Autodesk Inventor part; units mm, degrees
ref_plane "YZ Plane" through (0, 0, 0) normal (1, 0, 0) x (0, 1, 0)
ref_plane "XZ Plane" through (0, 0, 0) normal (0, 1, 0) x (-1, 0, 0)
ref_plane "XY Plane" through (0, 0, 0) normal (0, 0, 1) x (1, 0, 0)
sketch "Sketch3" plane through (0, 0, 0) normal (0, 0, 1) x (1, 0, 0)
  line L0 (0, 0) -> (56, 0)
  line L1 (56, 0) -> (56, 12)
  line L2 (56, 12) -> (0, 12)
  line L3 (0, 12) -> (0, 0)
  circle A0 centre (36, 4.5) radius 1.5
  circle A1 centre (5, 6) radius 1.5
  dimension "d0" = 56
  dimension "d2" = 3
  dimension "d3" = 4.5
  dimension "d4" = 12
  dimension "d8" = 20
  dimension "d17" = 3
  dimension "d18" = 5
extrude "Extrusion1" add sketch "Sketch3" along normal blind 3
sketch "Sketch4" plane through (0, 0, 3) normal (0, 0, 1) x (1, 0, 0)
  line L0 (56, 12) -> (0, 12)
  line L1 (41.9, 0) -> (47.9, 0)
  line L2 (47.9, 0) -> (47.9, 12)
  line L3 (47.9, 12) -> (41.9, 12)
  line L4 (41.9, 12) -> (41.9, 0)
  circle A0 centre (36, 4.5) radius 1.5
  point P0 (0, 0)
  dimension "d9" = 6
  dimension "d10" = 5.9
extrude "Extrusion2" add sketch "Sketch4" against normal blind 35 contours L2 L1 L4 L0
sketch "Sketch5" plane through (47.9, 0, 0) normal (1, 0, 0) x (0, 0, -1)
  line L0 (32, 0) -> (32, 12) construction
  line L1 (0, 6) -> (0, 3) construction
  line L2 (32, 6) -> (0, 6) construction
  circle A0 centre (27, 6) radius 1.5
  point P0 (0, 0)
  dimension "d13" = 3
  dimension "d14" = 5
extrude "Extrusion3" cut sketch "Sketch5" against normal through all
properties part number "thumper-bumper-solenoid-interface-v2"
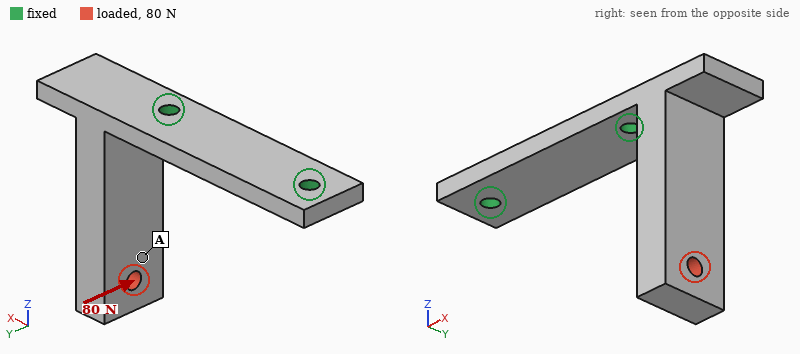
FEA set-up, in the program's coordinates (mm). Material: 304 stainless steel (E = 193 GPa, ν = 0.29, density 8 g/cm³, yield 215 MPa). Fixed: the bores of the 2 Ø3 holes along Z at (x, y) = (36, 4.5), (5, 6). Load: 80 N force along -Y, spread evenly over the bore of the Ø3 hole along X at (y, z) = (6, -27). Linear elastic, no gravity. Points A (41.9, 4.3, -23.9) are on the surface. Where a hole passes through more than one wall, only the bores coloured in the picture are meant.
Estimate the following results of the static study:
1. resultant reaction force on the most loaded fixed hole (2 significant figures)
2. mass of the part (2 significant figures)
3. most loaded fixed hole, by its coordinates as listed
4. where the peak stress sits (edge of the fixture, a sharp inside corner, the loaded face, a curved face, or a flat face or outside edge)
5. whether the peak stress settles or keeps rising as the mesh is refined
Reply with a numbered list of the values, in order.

1. 94 N
2. 34 g
3. (36, 4.5)
4. edge of the fixture
5. keeps rising
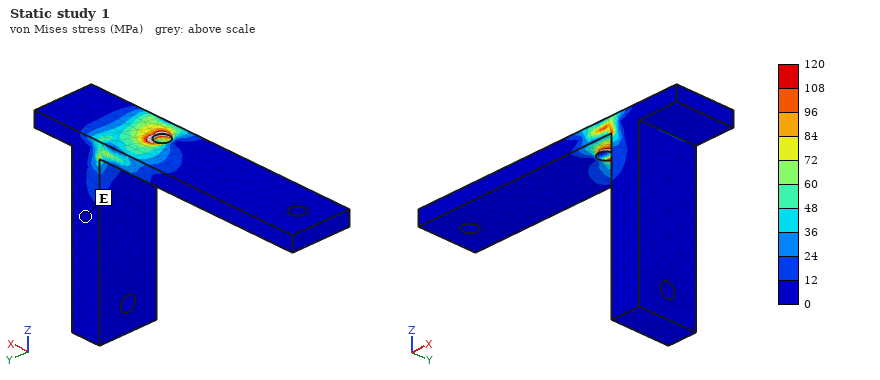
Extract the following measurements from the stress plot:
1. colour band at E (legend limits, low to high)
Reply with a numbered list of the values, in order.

1. 0 to 12 MPa
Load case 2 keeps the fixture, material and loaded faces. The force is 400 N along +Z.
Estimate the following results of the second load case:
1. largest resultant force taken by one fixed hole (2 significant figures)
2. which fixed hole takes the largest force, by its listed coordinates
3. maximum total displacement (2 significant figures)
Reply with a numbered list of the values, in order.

1. 410 N
2. (36, 4.5)
3. 100 µm
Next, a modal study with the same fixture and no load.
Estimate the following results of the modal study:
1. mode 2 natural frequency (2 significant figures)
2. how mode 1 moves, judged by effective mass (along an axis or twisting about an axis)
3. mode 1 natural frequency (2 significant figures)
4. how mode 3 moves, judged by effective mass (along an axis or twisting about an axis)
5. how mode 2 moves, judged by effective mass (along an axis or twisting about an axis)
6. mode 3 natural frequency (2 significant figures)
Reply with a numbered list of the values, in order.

1. 2100 Hz
2. along X
3. 1500 Hz
4. along Z
5. along Y
6. 8900 Hz
